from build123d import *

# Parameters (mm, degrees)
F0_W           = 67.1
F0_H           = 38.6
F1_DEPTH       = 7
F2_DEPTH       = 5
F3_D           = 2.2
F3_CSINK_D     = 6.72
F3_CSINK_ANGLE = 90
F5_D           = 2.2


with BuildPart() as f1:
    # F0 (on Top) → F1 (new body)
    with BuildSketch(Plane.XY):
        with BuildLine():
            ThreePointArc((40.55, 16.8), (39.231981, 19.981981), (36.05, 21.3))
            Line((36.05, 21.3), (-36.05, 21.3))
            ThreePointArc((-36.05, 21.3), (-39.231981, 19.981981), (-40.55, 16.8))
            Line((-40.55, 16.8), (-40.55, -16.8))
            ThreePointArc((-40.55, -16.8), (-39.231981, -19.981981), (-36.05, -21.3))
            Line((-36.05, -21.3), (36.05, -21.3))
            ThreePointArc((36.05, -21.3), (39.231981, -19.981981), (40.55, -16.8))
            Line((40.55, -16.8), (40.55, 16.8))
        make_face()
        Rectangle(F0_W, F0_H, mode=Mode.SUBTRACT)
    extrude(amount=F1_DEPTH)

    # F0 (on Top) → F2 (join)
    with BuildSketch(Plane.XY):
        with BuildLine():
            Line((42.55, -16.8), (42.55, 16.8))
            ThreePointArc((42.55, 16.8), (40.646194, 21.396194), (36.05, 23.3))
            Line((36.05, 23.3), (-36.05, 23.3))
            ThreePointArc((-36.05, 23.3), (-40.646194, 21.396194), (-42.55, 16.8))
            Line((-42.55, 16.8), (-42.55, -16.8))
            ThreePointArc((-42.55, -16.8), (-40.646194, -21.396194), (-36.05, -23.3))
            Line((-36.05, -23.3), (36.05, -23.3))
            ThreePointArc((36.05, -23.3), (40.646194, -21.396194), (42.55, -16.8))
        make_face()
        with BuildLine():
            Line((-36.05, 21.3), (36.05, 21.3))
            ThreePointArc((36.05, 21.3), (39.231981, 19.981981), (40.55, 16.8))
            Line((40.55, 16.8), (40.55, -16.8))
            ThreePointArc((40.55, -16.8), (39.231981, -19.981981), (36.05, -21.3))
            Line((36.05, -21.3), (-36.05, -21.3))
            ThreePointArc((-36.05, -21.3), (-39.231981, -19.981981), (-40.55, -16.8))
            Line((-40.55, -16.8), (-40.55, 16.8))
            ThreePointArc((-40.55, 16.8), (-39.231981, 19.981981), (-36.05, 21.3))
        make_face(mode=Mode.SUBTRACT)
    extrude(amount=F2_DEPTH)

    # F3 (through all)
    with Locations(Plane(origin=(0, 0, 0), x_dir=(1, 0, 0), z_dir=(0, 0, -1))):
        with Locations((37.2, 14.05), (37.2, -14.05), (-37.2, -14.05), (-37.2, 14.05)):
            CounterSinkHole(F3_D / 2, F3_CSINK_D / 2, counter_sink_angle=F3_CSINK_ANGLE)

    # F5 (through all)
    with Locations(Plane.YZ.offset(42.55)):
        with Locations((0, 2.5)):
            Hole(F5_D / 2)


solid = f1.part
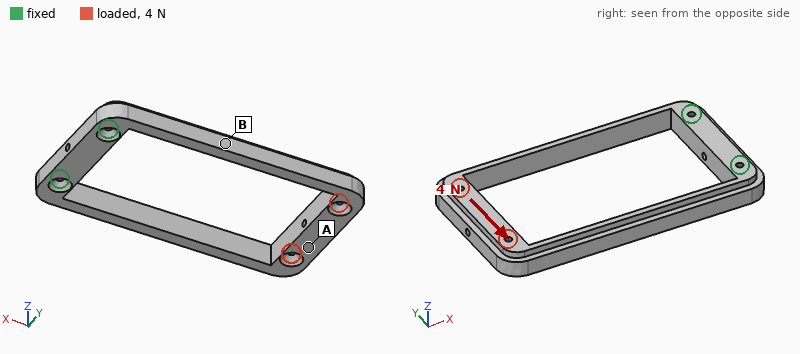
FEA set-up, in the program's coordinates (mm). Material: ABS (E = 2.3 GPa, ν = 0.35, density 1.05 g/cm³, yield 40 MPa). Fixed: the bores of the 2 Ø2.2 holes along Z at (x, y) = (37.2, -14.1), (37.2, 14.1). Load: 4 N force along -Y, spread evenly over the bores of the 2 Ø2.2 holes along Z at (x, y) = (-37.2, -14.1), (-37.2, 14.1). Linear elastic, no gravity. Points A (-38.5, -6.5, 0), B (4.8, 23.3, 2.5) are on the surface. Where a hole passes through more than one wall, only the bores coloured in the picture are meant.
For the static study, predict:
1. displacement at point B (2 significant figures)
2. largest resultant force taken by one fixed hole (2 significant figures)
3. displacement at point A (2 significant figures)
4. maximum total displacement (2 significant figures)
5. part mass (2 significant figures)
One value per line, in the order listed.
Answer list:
0.40 mm
8.4 N
0.97 mm
0.98 mm
8.5 g
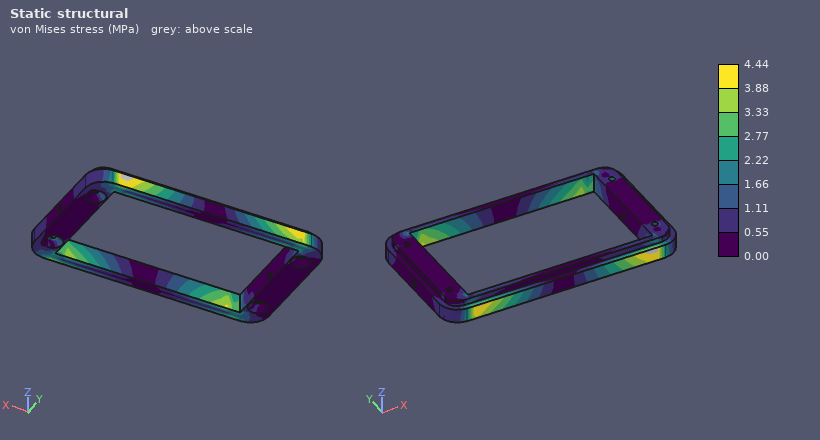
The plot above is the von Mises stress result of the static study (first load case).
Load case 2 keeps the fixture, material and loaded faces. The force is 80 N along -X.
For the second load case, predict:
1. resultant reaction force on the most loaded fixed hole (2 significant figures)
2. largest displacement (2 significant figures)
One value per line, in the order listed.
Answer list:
41 N
1.0 mm
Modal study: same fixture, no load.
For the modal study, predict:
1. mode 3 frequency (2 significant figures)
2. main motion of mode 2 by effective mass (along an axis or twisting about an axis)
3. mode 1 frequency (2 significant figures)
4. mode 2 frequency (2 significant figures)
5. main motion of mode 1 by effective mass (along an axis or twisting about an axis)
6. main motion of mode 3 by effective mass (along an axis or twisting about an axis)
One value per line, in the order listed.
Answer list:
360 Hz
along Y
140 Hz
170 Hz
along Z
twisting about X
